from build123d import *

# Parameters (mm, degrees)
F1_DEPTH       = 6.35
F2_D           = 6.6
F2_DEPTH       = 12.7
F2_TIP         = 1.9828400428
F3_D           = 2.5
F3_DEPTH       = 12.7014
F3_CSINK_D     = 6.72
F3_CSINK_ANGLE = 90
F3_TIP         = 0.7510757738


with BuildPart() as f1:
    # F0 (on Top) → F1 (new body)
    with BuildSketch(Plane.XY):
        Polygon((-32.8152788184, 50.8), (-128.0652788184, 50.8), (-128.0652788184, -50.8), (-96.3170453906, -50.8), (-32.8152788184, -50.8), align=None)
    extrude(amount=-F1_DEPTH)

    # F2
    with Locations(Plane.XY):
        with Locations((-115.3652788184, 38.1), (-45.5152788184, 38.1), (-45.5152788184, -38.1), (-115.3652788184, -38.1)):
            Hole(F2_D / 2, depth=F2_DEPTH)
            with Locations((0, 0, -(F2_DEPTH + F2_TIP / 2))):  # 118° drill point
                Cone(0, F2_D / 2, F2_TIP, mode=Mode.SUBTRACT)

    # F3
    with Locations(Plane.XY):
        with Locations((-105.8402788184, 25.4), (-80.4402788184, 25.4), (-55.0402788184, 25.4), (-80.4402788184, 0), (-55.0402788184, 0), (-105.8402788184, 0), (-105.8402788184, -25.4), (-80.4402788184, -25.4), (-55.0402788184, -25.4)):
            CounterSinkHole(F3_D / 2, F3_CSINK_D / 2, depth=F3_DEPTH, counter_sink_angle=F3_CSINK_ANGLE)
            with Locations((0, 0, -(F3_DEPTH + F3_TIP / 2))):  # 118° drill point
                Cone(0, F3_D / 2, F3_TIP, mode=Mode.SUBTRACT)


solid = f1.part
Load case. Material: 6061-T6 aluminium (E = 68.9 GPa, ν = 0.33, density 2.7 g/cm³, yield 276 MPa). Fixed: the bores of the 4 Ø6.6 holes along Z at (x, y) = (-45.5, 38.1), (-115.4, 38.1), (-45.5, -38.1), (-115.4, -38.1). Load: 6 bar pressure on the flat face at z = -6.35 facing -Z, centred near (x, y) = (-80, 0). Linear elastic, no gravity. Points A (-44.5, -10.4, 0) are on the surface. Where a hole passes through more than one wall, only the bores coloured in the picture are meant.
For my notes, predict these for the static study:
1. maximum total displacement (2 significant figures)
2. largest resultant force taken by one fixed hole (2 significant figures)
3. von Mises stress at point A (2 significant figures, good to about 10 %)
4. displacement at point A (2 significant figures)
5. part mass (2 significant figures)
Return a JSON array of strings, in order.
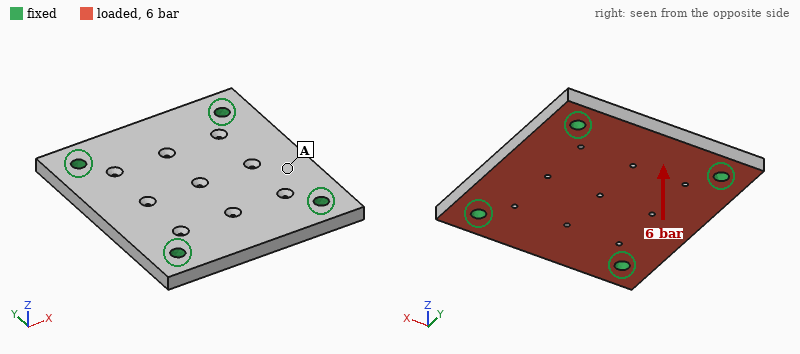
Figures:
["74 µm", "1.4 kN", "19 MPa", "40 µm", "160 g"]
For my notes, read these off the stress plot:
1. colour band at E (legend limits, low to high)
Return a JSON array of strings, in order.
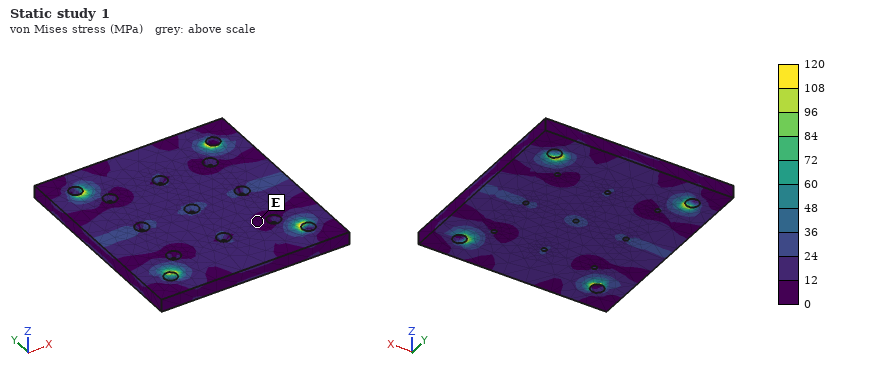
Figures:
["0 to 12 MPa"]
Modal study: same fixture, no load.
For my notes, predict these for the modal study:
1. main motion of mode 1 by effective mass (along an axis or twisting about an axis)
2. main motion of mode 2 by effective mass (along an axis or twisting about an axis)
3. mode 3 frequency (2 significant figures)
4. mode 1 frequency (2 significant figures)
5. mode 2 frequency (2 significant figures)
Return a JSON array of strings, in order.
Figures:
["along Z", "twisting about Y", "6700 Hz", "4300 Hz", "6200 Hz"]
